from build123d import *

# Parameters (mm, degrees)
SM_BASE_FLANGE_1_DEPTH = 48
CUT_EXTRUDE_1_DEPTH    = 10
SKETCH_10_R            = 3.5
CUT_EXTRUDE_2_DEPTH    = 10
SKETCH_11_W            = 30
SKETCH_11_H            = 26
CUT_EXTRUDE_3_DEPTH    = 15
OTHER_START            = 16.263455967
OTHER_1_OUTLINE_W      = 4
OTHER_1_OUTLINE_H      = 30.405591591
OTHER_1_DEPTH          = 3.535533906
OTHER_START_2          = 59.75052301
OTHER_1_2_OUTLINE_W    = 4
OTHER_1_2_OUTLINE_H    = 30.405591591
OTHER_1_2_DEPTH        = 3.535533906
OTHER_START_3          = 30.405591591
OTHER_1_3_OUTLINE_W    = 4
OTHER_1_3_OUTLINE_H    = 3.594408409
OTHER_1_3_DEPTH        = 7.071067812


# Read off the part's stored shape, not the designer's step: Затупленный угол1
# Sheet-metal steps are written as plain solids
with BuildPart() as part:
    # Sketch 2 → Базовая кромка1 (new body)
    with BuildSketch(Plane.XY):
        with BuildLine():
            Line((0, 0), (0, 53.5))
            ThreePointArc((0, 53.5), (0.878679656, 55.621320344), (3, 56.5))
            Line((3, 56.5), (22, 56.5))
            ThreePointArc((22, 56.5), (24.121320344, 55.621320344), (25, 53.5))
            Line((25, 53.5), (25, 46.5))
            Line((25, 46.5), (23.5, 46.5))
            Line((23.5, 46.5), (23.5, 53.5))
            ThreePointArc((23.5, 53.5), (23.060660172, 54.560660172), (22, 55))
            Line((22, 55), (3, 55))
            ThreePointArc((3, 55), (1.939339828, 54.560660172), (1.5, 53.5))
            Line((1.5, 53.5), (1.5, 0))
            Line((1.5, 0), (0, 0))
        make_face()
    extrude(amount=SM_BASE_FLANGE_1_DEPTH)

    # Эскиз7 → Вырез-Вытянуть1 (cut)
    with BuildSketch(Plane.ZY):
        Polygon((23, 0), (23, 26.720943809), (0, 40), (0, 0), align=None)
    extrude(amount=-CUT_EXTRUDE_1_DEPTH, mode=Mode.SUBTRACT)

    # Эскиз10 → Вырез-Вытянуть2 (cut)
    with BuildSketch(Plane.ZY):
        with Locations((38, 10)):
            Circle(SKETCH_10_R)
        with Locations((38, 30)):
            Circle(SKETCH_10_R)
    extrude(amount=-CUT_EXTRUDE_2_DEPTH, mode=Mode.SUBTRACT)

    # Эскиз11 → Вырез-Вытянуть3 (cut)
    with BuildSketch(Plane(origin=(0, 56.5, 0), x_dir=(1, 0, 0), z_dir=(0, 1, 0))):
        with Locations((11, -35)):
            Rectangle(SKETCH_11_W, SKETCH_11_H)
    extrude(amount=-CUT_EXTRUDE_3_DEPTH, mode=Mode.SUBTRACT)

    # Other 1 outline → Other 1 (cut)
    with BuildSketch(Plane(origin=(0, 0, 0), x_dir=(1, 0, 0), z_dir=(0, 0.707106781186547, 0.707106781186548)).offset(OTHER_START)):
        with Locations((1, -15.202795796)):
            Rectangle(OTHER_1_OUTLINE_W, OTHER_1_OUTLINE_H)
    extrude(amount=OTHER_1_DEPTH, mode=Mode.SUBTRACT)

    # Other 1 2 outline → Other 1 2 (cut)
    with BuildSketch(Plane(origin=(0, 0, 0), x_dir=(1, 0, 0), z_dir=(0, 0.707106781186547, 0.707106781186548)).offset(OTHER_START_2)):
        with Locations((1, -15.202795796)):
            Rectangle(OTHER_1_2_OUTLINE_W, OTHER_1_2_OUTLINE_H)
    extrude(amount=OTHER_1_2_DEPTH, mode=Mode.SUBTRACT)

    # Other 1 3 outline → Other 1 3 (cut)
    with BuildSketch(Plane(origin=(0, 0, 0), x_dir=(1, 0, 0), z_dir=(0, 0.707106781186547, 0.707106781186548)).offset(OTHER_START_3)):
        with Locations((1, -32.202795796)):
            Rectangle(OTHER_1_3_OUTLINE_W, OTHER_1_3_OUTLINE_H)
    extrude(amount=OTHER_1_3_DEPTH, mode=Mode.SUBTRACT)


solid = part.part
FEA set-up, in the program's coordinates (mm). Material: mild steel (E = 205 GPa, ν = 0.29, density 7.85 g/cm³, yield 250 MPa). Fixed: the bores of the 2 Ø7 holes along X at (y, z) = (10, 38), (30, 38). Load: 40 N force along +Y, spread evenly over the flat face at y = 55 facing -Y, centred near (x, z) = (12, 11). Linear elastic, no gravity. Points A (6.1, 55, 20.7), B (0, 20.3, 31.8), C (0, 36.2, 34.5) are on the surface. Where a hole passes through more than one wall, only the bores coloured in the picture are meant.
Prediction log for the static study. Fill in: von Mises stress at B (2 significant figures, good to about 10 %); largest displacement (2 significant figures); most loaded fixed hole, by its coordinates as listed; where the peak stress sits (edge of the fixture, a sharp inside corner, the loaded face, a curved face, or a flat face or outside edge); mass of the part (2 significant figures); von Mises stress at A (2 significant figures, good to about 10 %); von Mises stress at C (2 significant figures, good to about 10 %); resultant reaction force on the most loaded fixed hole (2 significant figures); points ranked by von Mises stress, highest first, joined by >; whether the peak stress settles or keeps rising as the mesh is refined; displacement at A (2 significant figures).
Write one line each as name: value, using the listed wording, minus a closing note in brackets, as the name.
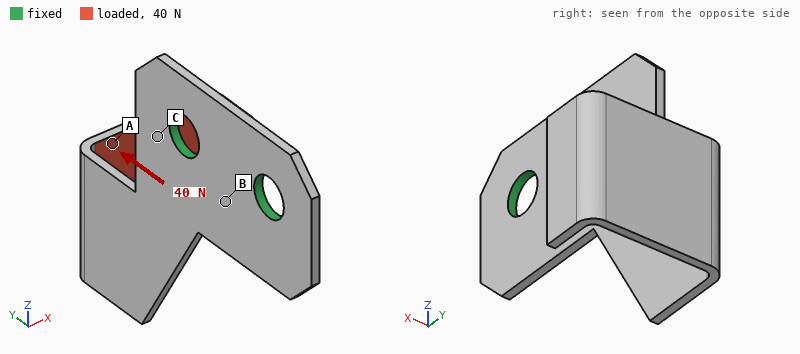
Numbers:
von Mises stress at B: 13 MPa
largest displacement: 0.45 mm
most loaded fixed hole, by its coordinates as listed: (10, 38)
where the peak stress sits: a sharp inside corner
mass of the part: 25 g
von Mises stress at A: 30 MPa
von Mises stress at C: 47 MPa
resultant reaction force on the most loaded fixed hole: 47 N
points ranked by von Mises stress, highest first, joined by >: C > A > B
whether the peak stress settles or keeps rising as the mesh is refined: keeps rising
displacement at A: 0.21 mm
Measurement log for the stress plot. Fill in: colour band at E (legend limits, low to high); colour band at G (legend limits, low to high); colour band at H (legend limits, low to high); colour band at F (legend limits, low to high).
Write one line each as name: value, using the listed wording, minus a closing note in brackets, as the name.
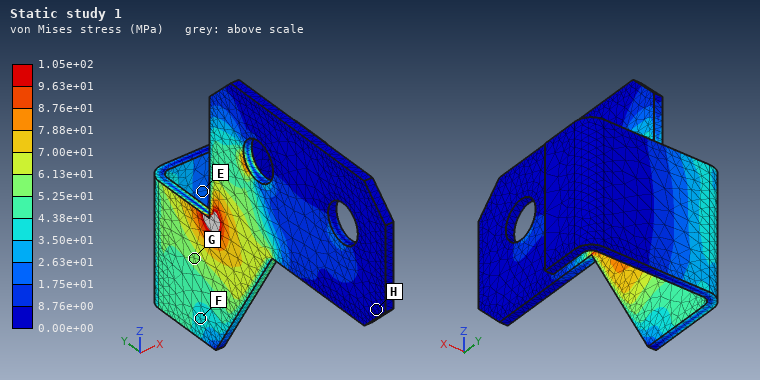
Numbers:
colour band at E: 1.75e+01 to 2.63e+01 MPa
colour band at G: 5.25e+01 to 6.13e+01 MPa
colour band at H: 0.00e+00 to 8.76e+00 MPa
colour band at F: 3.50e+01 to 4.38e+01 MPa
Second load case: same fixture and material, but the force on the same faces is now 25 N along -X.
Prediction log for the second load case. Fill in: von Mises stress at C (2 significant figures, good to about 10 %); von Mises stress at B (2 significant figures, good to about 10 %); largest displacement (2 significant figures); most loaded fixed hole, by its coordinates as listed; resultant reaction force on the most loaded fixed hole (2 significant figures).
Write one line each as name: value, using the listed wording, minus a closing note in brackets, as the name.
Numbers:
von Mises stress at C: 93 MPa
von Mises stress at B: 16 MPa
largest displacement: 0.59 mm
most loaded fixed hole, by its coordinates as listed: (30, 38)
resultant reaction force on the most loaded fixed hole: 37 N
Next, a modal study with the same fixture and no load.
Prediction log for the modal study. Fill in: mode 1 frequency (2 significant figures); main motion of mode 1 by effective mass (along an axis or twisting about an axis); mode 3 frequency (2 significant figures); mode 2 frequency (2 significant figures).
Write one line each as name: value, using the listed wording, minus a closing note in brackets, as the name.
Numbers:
mode 1 frequency: 340 Hz
main motion of mode 1 by effective mass: along X
mode 3 frequency: 1200 Hz
mode 2 frequency: 600 Hz
